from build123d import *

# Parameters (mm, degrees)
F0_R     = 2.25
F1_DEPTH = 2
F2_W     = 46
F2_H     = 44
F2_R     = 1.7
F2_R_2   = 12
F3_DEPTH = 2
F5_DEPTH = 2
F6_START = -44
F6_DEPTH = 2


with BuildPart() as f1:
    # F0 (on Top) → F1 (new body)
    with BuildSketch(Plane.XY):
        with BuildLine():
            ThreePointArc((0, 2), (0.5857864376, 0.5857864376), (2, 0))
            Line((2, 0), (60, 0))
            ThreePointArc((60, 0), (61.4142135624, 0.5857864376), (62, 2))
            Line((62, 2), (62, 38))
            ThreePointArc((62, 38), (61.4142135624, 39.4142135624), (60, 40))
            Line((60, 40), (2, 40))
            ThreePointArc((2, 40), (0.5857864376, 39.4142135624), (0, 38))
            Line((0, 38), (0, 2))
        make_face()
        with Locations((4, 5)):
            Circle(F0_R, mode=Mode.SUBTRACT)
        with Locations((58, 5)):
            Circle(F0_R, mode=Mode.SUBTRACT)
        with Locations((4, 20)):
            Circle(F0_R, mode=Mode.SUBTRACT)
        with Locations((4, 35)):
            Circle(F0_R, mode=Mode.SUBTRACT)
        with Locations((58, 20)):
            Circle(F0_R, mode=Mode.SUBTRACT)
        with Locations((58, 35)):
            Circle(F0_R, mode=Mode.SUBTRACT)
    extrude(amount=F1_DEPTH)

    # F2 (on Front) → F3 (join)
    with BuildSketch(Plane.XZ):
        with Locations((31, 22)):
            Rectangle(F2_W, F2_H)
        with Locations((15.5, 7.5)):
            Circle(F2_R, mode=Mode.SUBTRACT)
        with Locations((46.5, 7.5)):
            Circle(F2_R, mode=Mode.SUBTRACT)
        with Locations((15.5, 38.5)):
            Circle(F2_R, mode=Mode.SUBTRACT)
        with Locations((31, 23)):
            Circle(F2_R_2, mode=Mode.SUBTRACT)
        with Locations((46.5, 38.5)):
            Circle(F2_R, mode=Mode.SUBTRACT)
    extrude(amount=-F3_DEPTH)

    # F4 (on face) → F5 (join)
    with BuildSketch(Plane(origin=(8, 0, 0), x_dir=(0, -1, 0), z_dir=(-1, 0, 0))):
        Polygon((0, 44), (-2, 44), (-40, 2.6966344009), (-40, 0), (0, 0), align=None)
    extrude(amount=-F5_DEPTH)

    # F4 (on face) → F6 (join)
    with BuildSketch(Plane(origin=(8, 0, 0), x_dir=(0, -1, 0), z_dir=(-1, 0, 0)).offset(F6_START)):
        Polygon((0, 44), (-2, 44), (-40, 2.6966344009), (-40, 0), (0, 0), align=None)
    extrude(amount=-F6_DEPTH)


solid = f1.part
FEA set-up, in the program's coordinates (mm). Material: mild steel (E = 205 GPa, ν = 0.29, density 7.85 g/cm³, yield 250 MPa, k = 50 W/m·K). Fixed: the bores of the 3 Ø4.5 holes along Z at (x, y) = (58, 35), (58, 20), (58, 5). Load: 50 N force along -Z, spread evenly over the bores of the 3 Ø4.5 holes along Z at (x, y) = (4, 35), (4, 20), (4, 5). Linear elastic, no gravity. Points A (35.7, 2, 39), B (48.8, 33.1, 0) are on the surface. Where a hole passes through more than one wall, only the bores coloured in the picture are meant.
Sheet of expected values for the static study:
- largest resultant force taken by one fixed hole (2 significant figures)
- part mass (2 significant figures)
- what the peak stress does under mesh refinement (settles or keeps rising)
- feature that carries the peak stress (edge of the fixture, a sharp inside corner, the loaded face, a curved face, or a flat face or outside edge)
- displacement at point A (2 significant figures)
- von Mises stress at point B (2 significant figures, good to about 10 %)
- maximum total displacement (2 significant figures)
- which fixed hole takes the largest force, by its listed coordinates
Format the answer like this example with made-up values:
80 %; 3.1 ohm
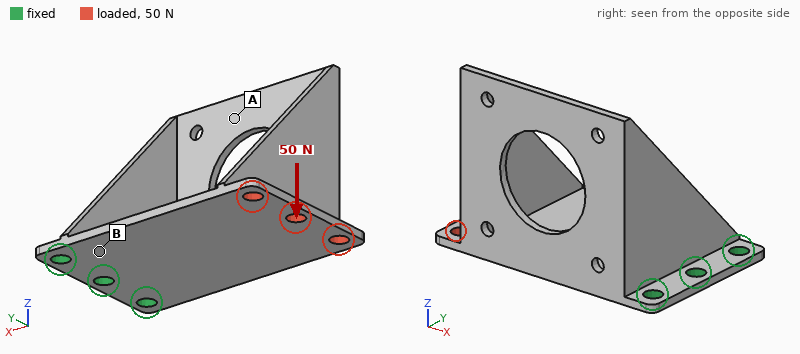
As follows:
45 N; 86 g; keeps rising; edge of the fixture; 0.13 mm; 38 MPa; 0.20 mm; (58, 20)
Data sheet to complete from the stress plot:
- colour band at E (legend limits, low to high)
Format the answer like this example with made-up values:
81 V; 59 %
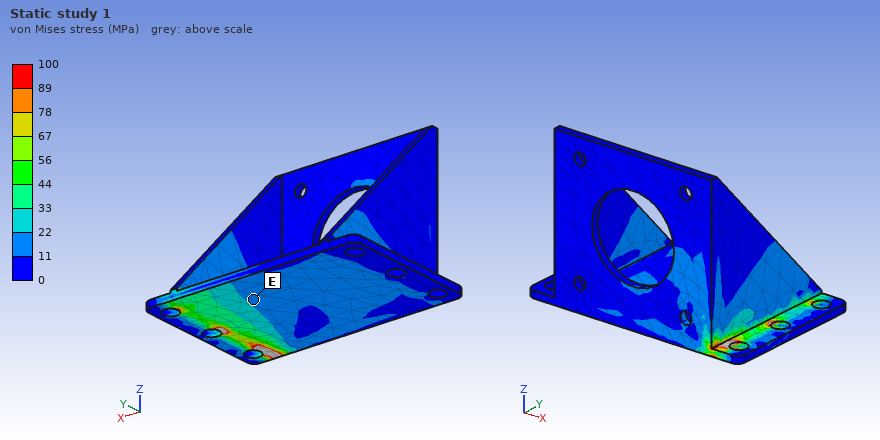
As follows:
11 to 22 MPa
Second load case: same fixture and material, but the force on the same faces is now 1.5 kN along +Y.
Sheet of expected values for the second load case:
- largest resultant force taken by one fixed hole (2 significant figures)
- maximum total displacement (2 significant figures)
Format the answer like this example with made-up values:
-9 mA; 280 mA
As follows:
2.6 kN; 63 µm
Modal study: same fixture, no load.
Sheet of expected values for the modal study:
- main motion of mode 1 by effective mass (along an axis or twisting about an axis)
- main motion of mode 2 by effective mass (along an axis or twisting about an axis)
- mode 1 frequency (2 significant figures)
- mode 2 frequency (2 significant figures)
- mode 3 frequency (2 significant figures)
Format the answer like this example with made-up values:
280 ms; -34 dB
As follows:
along Z; along Y; 460 Hz; 1000 Hz; 3500 Hz
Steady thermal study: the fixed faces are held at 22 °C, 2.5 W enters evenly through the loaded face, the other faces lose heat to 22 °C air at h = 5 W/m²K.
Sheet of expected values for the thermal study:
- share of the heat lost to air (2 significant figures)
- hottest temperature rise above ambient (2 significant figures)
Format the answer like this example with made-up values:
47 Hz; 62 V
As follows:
23 %; 25 K
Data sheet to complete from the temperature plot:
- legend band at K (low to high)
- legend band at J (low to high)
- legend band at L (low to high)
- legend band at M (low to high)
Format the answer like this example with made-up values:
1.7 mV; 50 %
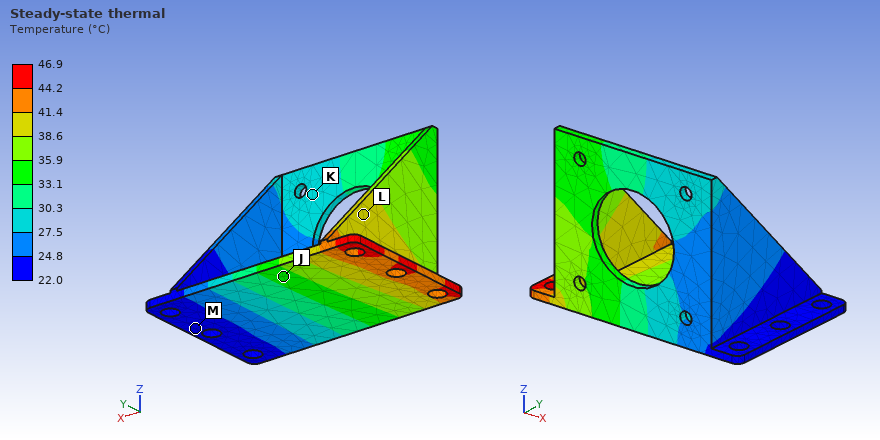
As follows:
27.5 to 30.3 °C; 33.1 to 35.9 °C; 38.6 to 41.4 °C; 22.0 to 24.8 °C
